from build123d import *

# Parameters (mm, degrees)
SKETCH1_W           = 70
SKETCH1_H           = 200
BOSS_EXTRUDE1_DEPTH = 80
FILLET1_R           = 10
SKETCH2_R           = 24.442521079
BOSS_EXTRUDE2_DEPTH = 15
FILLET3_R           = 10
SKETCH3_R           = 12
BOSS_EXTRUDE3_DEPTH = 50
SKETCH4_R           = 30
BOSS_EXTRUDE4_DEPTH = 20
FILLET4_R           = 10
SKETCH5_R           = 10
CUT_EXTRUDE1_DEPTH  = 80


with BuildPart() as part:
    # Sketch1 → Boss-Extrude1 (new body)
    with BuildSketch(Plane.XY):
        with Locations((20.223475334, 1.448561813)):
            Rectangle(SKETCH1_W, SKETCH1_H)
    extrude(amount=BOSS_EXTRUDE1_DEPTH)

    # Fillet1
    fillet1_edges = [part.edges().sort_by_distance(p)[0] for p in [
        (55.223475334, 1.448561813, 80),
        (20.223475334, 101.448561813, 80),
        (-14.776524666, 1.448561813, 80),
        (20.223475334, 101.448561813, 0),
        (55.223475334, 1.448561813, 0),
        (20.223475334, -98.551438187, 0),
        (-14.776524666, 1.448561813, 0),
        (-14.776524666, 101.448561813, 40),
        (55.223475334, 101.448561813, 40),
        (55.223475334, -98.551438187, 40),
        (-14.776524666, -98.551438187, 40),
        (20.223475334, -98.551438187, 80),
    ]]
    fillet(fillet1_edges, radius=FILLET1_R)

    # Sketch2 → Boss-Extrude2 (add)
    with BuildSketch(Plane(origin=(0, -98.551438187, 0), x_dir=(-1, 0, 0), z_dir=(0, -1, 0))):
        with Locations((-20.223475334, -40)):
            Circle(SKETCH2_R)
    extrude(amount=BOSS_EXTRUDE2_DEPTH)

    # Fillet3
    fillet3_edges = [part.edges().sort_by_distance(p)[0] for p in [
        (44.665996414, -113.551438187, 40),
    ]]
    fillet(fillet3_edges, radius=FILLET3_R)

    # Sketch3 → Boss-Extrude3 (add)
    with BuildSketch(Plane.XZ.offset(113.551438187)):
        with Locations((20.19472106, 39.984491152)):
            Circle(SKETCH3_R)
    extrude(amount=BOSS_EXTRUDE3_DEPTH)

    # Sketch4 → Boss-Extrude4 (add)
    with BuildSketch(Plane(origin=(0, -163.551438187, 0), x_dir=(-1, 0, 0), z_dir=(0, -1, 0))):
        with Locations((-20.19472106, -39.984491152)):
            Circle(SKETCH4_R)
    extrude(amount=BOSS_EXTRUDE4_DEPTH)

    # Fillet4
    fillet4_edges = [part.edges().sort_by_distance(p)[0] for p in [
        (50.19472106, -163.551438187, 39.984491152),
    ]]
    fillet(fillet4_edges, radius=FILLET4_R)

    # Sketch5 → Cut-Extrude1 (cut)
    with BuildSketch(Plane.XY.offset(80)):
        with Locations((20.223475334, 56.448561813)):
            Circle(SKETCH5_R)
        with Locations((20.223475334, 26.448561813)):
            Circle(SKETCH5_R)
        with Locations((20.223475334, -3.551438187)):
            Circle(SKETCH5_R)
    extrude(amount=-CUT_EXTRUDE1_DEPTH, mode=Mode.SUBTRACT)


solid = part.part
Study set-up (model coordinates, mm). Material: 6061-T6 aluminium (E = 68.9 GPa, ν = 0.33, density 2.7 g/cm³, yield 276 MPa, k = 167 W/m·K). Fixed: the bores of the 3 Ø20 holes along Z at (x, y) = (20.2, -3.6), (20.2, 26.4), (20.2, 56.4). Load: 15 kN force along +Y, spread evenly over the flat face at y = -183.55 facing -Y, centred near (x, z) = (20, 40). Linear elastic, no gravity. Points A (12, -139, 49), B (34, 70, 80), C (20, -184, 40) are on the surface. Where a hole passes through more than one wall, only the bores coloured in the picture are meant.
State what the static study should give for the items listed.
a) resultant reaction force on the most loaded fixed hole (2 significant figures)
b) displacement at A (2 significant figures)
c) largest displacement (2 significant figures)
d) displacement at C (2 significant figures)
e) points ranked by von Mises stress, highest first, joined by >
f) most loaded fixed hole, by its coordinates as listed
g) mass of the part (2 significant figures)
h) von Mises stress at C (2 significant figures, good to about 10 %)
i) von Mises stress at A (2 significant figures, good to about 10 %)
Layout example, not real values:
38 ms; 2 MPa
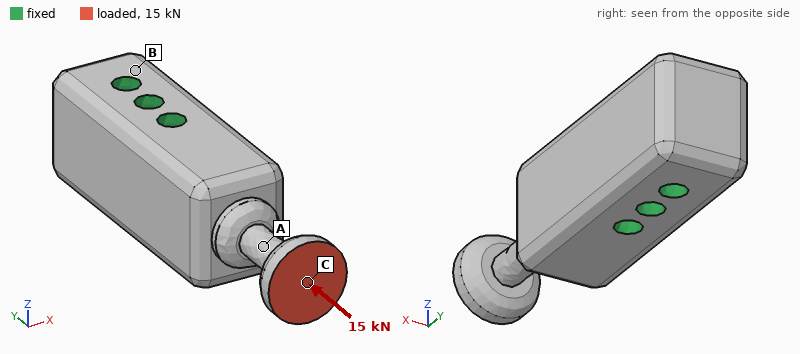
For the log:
12 kN; 22 µm; 42 µm; 36 µm; A > C > B; (20.2, -3.6); 3.0 kg; 19 MPa; 32 MPa
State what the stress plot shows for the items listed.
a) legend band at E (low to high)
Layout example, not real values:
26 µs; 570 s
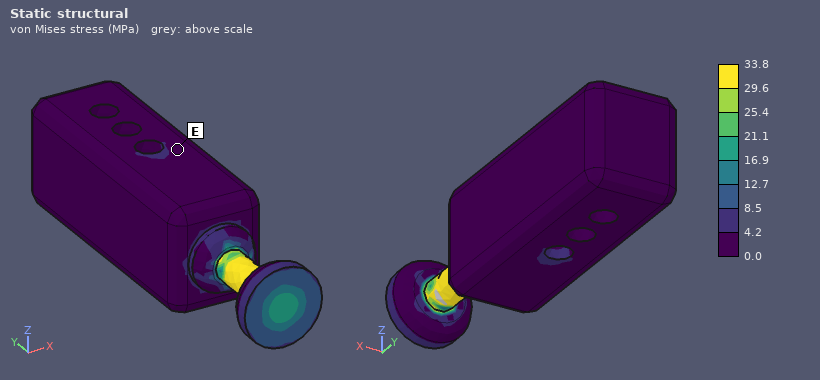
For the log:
0.0 to 4.2 MPa
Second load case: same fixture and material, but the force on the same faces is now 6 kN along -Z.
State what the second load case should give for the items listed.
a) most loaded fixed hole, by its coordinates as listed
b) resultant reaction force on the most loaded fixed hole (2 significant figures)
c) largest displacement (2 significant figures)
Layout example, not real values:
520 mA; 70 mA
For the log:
(20.2, -3.6); 8.1 kN; 0.95 mm
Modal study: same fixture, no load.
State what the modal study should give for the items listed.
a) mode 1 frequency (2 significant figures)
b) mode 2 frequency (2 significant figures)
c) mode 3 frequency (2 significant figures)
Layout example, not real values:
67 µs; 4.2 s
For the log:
1200 Hz; 1200 Hz; 2400 Hz
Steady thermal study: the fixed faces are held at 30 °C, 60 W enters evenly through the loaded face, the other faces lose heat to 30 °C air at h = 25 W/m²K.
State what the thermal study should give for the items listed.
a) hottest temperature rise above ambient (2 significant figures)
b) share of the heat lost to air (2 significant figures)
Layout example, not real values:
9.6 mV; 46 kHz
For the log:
51 K; 19 %
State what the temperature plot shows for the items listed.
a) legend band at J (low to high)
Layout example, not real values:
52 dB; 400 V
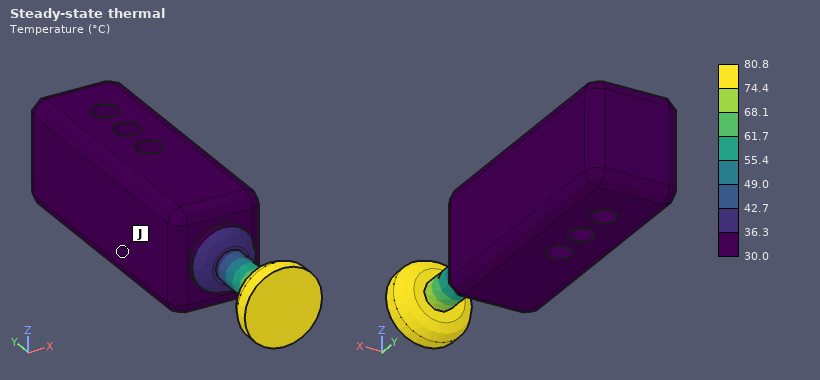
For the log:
30.0 to 36.3 °C
